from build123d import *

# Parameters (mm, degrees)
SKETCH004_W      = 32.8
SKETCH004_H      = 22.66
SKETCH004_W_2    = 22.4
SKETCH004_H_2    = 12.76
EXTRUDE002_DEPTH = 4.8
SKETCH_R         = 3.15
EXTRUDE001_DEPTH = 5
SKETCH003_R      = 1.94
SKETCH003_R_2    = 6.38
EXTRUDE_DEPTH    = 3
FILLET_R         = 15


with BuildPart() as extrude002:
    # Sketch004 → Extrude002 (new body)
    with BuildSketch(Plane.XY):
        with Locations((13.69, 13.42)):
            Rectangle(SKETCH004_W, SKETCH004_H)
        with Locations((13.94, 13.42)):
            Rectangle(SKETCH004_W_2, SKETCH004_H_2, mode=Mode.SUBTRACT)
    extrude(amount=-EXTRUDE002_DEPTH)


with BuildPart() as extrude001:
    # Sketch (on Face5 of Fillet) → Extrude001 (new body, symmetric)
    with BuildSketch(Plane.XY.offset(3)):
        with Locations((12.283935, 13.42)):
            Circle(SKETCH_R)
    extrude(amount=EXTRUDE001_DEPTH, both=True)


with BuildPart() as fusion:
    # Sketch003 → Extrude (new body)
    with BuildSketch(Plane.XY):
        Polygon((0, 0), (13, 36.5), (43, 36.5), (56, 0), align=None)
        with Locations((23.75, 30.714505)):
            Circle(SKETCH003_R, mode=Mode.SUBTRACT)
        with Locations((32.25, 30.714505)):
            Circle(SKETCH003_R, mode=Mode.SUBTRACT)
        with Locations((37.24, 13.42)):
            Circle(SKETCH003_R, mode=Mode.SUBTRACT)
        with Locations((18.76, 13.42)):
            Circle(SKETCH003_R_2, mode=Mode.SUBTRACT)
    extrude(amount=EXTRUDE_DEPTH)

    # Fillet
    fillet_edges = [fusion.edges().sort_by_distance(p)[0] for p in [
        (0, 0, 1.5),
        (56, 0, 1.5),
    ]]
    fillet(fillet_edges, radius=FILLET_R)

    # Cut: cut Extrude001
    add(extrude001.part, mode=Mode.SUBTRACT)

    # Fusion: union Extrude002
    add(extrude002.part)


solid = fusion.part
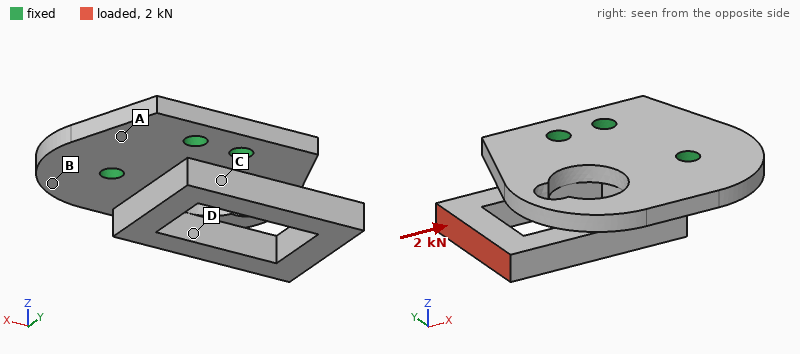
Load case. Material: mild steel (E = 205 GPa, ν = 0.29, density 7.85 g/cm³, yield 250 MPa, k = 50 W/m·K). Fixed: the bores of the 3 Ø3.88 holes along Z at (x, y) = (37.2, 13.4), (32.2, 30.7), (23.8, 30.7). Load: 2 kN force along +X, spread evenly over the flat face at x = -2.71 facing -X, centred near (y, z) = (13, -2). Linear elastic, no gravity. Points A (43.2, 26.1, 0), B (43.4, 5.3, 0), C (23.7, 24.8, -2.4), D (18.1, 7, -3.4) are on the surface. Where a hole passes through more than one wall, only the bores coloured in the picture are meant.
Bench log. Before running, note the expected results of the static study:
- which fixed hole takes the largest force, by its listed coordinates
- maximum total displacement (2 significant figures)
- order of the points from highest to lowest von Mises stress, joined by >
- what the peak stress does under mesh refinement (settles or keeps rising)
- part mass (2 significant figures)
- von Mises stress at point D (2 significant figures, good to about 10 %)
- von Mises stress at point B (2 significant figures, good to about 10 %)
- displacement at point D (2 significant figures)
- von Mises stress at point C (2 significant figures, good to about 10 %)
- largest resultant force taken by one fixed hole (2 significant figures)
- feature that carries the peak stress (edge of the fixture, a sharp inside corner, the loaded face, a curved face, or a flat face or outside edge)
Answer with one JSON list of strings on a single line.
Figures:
["(37.2, 13.4)", "83 µm", "C > D > B > A", "keeps rising", "45 g", "43 MPa", "26 MPa", "34 µm", "66 MPa", "1.5 kN", "edge of the fixture"]
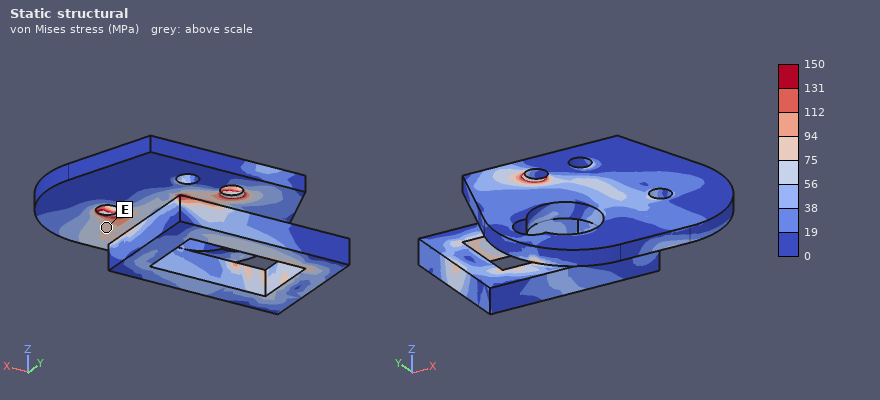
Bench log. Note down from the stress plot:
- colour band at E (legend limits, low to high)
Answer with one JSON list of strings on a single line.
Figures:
["75 to 94 MPa"]
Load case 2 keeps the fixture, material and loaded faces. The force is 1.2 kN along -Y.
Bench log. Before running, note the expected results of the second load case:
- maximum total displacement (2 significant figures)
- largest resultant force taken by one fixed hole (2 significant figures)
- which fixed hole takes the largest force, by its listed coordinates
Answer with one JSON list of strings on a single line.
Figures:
["56 µm", "1.7 kN", "(23.8, 30.7)"]
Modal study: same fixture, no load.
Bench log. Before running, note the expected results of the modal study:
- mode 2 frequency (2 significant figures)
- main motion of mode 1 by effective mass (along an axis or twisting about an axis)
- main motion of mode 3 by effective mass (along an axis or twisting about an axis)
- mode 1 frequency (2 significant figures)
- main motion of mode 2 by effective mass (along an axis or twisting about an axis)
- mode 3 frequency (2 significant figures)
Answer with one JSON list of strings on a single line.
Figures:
["9100 Hz", "along Z", "along Y", "3000 Hz", "twisting about X", "11 kHz"]
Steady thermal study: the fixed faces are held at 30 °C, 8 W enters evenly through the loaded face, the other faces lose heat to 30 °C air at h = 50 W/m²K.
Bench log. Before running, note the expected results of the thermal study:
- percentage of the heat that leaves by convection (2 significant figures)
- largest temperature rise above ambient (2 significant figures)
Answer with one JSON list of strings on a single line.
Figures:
["35 %", "61 K"]
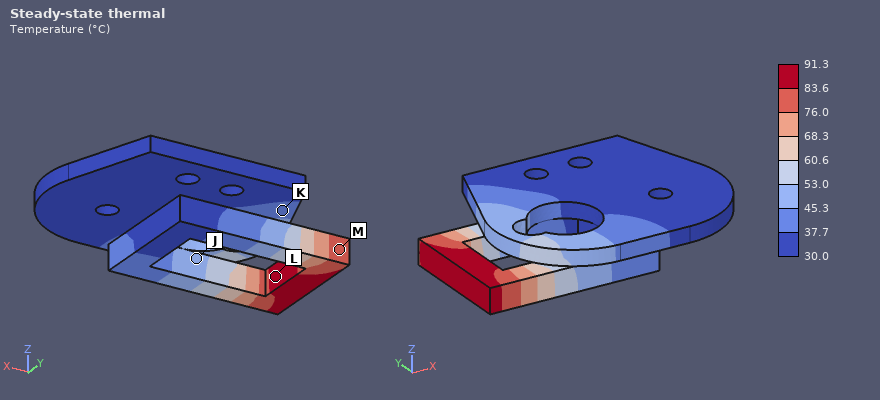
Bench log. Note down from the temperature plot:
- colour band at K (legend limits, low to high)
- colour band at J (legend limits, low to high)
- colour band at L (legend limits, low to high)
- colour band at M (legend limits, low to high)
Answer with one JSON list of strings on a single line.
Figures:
["37.7 to 45.3 °C", "45.3 to 53.0 °C", "83.6 to 91.3 °C", "76.0 to 83.6 °C"]
